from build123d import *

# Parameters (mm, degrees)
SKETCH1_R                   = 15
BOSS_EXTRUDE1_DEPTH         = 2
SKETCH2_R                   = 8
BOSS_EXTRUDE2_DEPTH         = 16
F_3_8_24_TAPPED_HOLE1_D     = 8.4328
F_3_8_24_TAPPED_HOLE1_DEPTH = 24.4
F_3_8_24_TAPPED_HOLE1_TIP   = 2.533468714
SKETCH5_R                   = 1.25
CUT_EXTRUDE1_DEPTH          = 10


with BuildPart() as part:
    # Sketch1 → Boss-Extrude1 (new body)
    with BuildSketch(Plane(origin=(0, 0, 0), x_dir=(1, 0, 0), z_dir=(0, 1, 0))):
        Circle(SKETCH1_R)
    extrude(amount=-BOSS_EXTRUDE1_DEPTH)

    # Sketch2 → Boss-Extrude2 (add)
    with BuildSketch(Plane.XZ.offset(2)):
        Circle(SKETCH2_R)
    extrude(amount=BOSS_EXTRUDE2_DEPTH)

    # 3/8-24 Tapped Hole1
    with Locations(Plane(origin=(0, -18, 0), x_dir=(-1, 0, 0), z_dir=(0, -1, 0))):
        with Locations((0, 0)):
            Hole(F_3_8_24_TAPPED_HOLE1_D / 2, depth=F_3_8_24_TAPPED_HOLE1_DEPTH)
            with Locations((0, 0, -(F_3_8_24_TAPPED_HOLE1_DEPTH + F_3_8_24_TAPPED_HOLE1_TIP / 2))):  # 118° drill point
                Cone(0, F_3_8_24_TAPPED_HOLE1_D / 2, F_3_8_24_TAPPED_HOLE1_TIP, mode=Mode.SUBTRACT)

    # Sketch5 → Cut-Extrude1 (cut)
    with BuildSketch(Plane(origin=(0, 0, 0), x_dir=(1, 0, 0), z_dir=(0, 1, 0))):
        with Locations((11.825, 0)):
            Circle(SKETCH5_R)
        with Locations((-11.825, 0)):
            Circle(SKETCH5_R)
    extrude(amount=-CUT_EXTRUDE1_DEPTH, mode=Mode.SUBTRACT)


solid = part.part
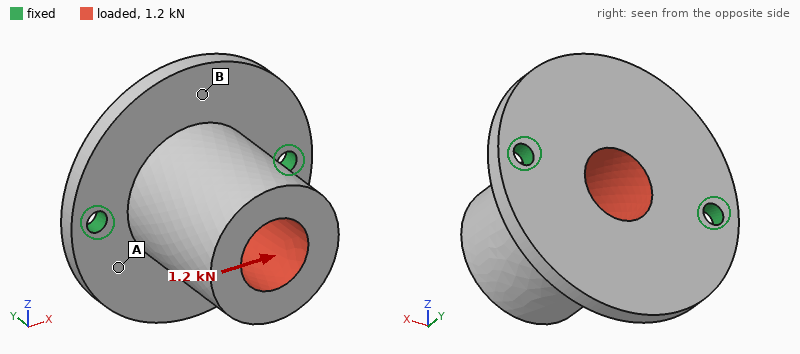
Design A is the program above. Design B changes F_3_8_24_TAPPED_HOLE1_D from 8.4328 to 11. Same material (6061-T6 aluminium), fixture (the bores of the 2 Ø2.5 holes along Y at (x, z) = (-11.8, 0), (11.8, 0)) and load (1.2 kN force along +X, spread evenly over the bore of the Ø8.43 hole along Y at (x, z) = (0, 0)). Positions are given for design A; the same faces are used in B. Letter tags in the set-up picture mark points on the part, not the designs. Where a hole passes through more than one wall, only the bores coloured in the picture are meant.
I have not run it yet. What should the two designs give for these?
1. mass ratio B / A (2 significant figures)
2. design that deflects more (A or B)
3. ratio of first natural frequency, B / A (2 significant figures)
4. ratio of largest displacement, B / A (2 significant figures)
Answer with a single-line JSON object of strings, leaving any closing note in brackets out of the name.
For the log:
{"mass ratio B / A": "0.80", "design that deflects more": "B", "ratio of first natural frequency, B / A": "1.1", "ratio of largest displacement, B / A": "1.1"}
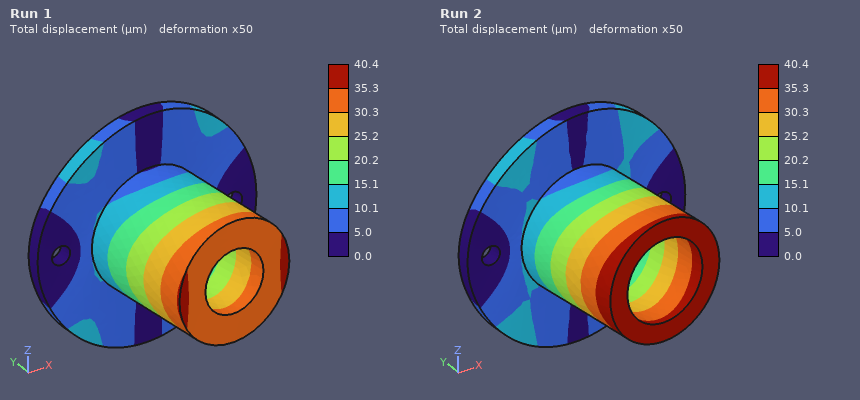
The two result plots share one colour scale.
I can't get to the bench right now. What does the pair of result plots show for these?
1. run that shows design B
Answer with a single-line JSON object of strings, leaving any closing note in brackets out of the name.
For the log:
{"run that shows design B": "Run 2"}
